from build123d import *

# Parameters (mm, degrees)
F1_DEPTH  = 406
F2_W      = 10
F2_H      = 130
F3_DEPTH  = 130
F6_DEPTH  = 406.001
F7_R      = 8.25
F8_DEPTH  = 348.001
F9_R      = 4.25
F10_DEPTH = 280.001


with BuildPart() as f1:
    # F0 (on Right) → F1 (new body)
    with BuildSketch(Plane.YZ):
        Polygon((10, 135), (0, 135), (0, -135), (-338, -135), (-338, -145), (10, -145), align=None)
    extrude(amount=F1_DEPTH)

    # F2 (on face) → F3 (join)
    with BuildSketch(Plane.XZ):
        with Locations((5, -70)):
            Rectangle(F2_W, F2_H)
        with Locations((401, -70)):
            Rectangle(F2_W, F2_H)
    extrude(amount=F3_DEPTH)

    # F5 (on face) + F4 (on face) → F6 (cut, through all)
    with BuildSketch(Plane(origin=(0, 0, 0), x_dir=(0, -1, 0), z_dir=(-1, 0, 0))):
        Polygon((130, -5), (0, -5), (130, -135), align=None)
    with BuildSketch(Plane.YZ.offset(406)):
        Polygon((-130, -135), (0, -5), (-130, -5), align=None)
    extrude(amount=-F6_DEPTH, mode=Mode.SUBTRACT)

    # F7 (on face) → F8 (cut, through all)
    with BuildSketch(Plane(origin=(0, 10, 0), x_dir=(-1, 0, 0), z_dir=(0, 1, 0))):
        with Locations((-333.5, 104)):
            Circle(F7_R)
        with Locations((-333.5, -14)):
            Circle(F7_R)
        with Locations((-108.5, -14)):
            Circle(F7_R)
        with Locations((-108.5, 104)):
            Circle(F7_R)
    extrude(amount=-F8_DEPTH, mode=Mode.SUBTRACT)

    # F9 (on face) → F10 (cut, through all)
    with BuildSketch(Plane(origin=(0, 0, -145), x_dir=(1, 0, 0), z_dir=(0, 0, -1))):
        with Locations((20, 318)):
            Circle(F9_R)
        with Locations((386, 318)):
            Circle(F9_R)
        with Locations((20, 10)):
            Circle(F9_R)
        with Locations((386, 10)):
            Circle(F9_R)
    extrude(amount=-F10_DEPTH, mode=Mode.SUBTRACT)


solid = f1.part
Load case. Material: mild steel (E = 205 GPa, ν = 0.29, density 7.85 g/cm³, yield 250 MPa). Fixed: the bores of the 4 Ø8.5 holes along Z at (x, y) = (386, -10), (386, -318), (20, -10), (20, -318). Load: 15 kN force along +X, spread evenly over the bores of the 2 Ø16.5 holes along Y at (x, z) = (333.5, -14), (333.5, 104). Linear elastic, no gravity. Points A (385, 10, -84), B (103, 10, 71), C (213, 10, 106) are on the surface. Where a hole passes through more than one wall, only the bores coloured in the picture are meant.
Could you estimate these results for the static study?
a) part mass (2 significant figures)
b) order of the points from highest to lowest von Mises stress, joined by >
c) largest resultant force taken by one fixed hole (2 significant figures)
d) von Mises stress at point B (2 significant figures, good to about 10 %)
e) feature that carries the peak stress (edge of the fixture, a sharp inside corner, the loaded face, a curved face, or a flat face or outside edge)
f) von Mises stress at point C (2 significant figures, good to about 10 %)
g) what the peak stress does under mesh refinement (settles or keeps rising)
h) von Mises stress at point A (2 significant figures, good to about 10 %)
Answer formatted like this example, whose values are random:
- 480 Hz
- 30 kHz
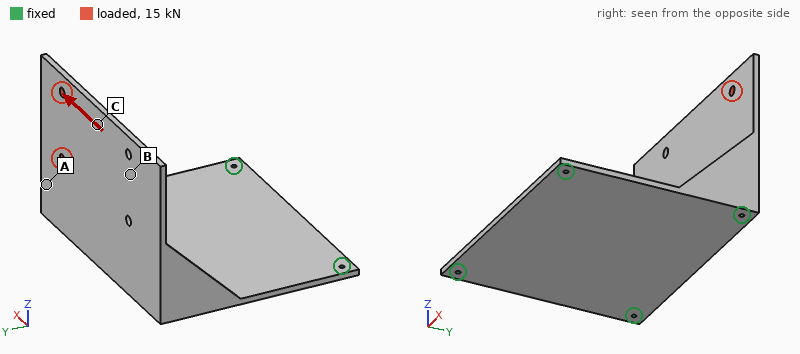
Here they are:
- 21 kg
- A > C > B
- 10 kN
- 2.5 MPa
- edge of the fixture
- 5.1 MPa
- keeps rising
- 8.4 MPa
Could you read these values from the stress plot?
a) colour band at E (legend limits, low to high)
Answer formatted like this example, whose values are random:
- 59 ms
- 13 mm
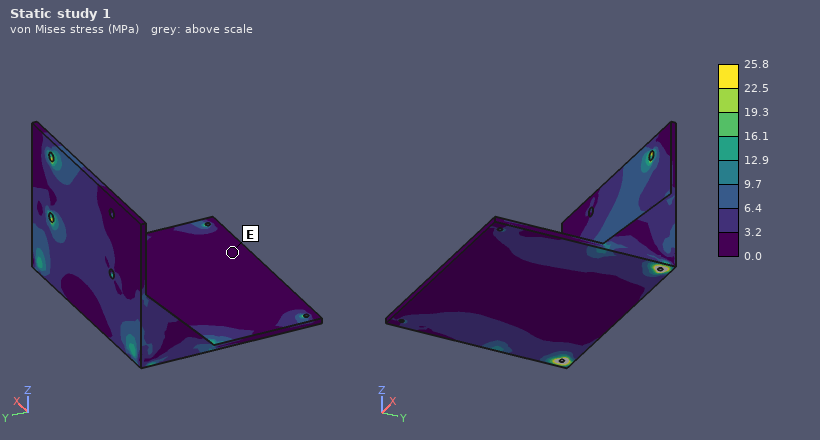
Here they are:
- 0.0 to 3.2 MPa
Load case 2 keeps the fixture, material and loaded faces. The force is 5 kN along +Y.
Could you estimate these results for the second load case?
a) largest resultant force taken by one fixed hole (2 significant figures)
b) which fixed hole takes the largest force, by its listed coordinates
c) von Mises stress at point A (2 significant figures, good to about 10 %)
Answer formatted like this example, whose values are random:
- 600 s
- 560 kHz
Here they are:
- 3.0 kN
- (386, -10)
- 47 MPa
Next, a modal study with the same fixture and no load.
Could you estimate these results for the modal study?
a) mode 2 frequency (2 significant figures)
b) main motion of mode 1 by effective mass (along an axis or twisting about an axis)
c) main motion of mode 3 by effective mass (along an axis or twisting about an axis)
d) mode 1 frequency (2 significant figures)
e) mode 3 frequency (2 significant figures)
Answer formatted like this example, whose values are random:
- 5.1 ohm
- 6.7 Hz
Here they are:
- 290 Hz
- along Y
- along Z
- 140 Hz
- 320 Hz
